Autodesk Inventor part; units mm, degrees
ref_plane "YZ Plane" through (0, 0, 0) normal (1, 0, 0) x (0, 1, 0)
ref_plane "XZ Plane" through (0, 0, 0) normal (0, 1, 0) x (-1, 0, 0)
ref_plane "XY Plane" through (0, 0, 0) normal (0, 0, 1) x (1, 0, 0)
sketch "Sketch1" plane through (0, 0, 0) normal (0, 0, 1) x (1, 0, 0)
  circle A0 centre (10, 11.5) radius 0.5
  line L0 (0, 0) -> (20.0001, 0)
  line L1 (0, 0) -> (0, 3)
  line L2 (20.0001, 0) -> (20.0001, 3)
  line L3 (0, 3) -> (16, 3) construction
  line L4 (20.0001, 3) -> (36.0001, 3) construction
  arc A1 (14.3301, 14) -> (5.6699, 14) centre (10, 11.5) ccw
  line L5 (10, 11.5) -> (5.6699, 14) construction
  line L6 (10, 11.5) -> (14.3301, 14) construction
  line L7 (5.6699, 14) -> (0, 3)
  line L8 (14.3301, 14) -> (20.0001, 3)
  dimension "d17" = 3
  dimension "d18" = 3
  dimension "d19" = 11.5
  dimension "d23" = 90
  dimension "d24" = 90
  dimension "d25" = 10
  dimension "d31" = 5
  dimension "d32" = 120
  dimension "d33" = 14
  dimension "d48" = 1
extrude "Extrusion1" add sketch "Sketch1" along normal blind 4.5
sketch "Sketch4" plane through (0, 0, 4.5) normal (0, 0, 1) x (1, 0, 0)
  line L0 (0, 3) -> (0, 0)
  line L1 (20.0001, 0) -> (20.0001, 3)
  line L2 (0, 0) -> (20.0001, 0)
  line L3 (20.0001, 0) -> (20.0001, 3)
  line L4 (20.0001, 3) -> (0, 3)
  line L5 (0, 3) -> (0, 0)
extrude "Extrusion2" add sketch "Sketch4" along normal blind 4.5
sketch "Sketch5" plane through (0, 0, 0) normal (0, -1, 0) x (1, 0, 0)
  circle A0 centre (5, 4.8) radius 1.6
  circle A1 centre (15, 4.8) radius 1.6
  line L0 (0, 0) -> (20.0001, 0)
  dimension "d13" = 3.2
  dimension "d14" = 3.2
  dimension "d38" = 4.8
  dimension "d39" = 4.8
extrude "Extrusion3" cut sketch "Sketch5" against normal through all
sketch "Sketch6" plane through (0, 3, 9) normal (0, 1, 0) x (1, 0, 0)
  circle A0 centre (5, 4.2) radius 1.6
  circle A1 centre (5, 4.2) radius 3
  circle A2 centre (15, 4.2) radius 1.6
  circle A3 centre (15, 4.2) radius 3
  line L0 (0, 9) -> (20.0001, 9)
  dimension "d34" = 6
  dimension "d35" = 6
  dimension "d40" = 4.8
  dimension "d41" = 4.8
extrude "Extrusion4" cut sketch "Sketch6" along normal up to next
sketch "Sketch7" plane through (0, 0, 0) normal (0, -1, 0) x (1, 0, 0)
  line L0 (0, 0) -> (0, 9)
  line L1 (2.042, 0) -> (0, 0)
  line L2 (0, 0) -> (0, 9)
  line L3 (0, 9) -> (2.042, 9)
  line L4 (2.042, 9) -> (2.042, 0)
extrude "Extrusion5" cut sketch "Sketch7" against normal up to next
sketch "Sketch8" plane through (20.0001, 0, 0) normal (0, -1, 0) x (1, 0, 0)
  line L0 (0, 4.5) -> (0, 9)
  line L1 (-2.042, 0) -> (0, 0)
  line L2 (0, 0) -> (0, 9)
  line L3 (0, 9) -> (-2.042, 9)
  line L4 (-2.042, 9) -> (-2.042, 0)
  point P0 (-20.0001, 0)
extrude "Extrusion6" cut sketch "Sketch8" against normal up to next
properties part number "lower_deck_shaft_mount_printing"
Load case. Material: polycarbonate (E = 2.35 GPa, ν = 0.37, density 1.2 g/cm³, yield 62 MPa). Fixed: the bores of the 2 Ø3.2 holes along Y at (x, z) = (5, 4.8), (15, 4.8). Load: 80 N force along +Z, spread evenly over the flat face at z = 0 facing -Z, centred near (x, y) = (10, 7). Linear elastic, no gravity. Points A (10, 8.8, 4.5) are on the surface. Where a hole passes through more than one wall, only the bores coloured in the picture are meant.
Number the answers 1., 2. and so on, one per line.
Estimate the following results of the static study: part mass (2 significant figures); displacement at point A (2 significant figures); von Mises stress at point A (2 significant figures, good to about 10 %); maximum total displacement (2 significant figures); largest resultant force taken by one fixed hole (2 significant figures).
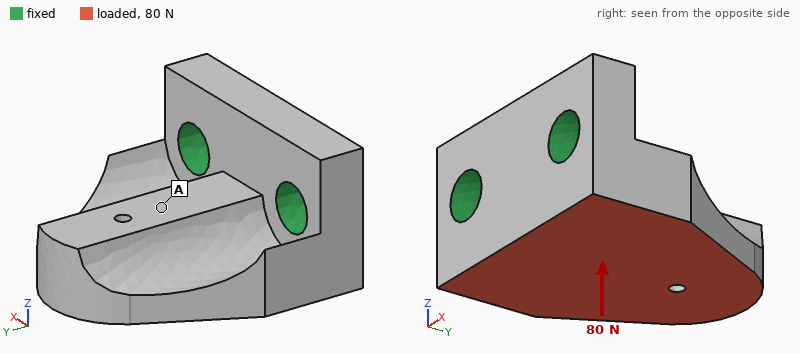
1. 1.1 g
2. 0.12 mm
3. 4.2 MPa
4. 0.28 mm
5. 41 N
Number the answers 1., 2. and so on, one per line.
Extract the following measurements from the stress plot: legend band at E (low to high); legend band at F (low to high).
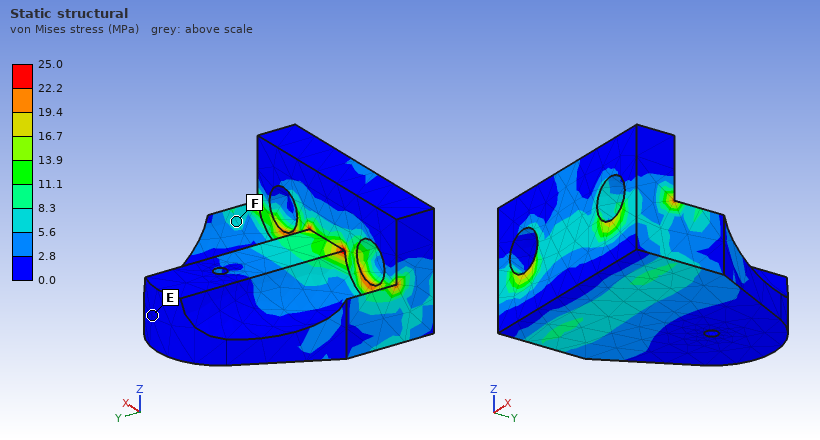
1. 0.0 to 2.8 MPa
2. 5.6 to 8.3 MPa
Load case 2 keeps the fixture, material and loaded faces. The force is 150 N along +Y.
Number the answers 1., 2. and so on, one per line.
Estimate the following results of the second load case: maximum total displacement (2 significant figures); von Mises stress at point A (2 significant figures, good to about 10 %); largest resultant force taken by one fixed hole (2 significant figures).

1. 0.26 mm
2. 2.8 MPa
3. 75 N
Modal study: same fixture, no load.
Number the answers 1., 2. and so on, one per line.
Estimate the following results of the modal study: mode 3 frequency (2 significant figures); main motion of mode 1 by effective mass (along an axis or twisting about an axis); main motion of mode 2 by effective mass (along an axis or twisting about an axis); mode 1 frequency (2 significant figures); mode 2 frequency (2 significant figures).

1. 12 kHz
2. along Z
3. along X
4. 3800 Hz
5. 8000 Hz
